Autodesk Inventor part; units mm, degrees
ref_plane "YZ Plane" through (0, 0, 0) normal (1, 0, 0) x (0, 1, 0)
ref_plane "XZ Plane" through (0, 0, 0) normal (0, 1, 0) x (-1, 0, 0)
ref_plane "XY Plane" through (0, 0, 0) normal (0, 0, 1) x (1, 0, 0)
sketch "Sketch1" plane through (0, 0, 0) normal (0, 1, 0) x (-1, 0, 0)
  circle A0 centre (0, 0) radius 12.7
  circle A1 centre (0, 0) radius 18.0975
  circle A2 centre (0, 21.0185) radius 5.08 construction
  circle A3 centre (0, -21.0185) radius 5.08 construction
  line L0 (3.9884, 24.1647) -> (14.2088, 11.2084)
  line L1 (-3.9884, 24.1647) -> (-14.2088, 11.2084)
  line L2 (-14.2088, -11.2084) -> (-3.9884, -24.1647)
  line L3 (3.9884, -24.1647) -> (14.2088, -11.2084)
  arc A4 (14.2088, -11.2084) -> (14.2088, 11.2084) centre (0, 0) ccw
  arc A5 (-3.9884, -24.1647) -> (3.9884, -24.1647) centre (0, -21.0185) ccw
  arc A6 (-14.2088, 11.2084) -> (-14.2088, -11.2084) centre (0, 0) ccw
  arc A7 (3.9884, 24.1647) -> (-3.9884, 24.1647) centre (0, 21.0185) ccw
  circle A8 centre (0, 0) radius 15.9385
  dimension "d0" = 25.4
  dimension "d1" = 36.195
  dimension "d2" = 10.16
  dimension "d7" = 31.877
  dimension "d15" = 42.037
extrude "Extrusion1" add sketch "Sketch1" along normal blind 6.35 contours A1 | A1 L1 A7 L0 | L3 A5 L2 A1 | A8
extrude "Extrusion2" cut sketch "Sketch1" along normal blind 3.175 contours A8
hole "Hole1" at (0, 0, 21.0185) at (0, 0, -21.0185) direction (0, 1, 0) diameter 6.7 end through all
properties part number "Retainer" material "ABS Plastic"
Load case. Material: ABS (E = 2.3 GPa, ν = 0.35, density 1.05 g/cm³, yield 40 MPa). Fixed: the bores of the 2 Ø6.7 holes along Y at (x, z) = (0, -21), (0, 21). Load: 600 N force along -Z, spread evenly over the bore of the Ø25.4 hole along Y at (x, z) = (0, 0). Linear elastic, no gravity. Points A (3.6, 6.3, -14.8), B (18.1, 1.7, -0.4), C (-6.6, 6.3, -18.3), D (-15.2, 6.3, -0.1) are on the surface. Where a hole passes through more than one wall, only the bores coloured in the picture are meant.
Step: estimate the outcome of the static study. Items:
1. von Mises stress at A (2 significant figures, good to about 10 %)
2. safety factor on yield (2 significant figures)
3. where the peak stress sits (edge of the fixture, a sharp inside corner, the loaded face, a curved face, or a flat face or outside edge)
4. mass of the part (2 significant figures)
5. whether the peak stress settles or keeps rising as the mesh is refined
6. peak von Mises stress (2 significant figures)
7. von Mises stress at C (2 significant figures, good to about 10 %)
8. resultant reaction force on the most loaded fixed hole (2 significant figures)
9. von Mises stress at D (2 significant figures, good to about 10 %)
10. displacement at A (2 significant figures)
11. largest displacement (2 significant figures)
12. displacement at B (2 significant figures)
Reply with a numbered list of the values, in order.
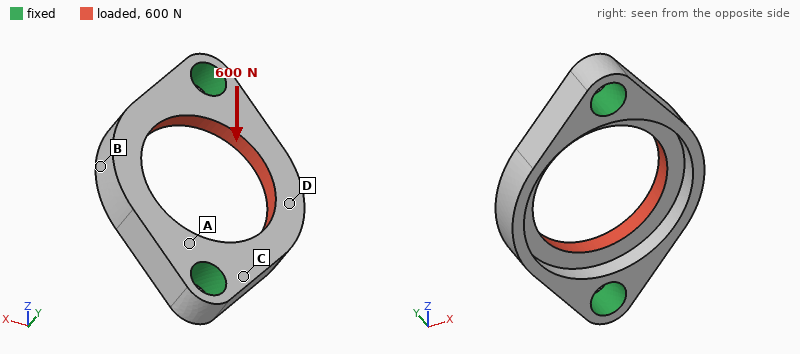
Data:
1. 6.2 MPa
2. 2.8
3. the loaded face
4. 3.5 g
5. settles
6. 14 MPa
7. 7.1 MPa
8. 300 N
9. 2.7 MPa
10. 15 µm
11. 94 µm
12. 54 µm
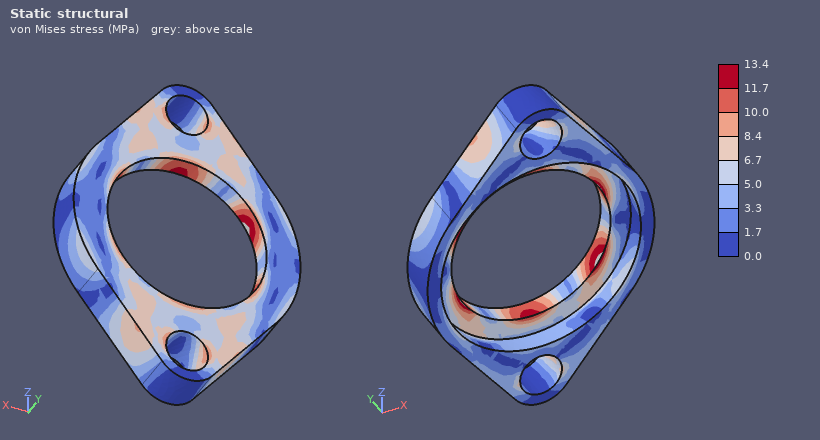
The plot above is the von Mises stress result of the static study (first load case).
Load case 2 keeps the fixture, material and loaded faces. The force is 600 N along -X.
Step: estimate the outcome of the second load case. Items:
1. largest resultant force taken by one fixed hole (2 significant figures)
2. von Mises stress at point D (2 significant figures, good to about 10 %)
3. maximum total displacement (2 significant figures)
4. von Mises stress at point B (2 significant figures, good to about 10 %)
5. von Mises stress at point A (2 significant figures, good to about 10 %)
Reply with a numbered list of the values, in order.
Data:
1. 300 N
2. 6.0 MPa
3. 0.15 mm
4. 3.9 MPa
5. 8.3 MPa
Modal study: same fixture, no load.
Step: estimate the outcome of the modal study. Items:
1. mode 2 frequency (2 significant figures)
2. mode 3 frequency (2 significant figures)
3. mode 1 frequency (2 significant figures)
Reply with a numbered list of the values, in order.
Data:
1. 3600 Hz
2. 7000 Hz
3. 3400 Hz
